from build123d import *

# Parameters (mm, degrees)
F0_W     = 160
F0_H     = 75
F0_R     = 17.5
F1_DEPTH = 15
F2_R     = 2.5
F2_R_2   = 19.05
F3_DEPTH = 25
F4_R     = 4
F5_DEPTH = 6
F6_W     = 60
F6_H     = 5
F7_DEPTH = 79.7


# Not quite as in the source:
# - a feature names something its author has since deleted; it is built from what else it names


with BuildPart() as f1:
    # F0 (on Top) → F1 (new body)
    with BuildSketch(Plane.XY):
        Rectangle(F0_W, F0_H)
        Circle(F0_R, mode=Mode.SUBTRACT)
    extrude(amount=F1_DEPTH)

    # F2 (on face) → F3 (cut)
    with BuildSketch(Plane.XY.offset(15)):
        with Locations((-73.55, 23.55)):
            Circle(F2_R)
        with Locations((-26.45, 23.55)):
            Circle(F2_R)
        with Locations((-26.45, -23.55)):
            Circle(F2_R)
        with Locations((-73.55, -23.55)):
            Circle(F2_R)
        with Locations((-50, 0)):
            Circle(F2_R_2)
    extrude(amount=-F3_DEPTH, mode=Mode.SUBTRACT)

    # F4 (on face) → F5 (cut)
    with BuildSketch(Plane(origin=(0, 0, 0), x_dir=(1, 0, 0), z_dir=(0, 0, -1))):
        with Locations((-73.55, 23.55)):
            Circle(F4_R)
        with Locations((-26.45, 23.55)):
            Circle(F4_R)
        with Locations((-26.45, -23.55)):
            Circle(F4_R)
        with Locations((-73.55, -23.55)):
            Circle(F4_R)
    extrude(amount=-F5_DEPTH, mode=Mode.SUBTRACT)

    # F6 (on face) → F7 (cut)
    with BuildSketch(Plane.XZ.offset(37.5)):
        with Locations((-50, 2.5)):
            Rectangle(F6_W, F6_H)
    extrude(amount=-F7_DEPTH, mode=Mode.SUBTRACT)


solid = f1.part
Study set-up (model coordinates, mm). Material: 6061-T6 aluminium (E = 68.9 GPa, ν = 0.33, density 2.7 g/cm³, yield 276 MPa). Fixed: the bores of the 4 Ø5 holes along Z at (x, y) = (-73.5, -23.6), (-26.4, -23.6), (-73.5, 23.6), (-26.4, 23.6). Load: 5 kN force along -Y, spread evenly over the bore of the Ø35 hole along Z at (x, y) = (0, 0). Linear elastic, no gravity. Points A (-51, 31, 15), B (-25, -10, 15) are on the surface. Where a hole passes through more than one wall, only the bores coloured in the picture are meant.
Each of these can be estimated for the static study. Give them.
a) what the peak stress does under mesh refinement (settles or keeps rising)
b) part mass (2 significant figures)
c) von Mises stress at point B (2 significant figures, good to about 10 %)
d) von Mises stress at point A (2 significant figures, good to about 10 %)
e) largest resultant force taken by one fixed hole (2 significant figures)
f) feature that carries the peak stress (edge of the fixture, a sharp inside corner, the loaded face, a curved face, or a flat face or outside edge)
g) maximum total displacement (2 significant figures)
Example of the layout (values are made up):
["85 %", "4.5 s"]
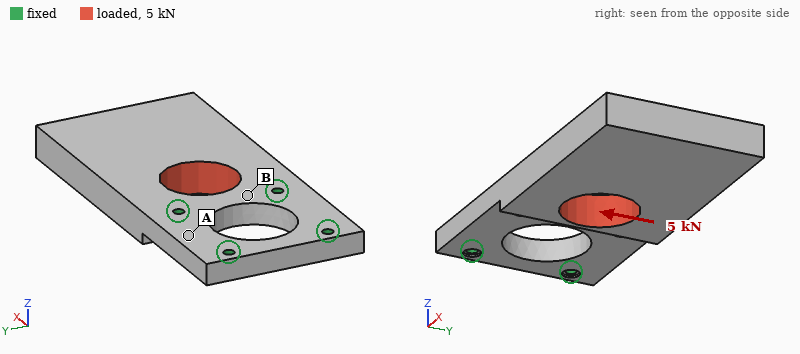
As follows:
["keeps rising", "350 g", "14 MPa", "5.3 MPa", "3.2 kN", "edge of the fixture", "38 µm"]
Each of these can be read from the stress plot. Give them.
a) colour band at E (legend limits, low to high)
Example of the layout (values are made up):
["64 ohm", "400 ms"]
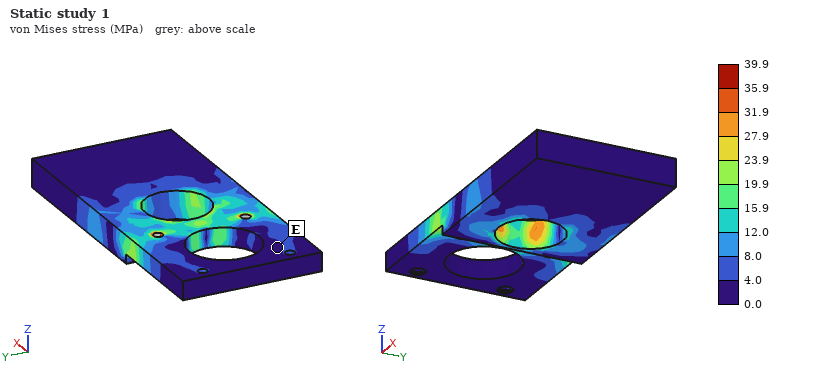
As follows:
["0.0 to 4.0 MPa"]
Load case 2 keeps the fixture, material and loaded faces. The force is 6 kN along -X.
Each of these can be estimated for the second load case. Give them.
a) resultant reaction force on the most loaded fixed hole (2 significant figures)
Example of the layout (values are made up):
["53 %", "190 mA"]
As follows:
["2.8 kN"]
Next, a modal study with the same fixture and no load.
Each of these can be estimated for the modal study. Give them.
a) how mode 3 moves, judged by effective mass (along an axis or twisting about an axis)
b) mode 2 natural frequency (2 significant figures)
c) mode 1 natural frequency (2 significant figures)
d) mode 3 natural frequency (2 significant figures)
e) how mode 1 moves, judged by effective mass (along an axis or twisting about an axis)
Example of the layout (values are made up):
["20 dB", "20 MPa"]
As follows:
["along Y", "2300 Hz", "620 Hz", "2700 Hz", "along Z"]
